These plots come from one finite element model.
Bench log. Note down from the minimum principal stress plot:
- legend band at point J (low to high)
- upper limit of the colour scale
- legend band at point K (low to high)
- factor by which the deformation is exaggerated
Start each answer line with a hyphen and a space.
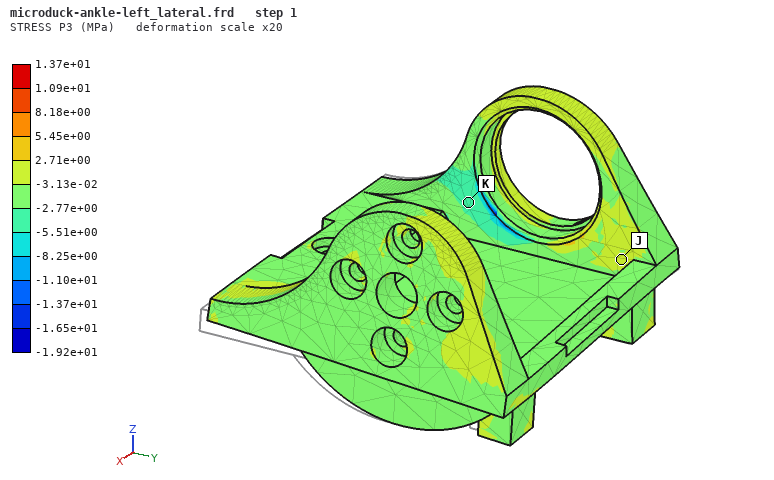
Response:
- -3.13e-02 to 2.71e+00 MPa
- 1.37e+01 MPa
- -5.51e+00 to -2.77e+00 MPa
- 20
